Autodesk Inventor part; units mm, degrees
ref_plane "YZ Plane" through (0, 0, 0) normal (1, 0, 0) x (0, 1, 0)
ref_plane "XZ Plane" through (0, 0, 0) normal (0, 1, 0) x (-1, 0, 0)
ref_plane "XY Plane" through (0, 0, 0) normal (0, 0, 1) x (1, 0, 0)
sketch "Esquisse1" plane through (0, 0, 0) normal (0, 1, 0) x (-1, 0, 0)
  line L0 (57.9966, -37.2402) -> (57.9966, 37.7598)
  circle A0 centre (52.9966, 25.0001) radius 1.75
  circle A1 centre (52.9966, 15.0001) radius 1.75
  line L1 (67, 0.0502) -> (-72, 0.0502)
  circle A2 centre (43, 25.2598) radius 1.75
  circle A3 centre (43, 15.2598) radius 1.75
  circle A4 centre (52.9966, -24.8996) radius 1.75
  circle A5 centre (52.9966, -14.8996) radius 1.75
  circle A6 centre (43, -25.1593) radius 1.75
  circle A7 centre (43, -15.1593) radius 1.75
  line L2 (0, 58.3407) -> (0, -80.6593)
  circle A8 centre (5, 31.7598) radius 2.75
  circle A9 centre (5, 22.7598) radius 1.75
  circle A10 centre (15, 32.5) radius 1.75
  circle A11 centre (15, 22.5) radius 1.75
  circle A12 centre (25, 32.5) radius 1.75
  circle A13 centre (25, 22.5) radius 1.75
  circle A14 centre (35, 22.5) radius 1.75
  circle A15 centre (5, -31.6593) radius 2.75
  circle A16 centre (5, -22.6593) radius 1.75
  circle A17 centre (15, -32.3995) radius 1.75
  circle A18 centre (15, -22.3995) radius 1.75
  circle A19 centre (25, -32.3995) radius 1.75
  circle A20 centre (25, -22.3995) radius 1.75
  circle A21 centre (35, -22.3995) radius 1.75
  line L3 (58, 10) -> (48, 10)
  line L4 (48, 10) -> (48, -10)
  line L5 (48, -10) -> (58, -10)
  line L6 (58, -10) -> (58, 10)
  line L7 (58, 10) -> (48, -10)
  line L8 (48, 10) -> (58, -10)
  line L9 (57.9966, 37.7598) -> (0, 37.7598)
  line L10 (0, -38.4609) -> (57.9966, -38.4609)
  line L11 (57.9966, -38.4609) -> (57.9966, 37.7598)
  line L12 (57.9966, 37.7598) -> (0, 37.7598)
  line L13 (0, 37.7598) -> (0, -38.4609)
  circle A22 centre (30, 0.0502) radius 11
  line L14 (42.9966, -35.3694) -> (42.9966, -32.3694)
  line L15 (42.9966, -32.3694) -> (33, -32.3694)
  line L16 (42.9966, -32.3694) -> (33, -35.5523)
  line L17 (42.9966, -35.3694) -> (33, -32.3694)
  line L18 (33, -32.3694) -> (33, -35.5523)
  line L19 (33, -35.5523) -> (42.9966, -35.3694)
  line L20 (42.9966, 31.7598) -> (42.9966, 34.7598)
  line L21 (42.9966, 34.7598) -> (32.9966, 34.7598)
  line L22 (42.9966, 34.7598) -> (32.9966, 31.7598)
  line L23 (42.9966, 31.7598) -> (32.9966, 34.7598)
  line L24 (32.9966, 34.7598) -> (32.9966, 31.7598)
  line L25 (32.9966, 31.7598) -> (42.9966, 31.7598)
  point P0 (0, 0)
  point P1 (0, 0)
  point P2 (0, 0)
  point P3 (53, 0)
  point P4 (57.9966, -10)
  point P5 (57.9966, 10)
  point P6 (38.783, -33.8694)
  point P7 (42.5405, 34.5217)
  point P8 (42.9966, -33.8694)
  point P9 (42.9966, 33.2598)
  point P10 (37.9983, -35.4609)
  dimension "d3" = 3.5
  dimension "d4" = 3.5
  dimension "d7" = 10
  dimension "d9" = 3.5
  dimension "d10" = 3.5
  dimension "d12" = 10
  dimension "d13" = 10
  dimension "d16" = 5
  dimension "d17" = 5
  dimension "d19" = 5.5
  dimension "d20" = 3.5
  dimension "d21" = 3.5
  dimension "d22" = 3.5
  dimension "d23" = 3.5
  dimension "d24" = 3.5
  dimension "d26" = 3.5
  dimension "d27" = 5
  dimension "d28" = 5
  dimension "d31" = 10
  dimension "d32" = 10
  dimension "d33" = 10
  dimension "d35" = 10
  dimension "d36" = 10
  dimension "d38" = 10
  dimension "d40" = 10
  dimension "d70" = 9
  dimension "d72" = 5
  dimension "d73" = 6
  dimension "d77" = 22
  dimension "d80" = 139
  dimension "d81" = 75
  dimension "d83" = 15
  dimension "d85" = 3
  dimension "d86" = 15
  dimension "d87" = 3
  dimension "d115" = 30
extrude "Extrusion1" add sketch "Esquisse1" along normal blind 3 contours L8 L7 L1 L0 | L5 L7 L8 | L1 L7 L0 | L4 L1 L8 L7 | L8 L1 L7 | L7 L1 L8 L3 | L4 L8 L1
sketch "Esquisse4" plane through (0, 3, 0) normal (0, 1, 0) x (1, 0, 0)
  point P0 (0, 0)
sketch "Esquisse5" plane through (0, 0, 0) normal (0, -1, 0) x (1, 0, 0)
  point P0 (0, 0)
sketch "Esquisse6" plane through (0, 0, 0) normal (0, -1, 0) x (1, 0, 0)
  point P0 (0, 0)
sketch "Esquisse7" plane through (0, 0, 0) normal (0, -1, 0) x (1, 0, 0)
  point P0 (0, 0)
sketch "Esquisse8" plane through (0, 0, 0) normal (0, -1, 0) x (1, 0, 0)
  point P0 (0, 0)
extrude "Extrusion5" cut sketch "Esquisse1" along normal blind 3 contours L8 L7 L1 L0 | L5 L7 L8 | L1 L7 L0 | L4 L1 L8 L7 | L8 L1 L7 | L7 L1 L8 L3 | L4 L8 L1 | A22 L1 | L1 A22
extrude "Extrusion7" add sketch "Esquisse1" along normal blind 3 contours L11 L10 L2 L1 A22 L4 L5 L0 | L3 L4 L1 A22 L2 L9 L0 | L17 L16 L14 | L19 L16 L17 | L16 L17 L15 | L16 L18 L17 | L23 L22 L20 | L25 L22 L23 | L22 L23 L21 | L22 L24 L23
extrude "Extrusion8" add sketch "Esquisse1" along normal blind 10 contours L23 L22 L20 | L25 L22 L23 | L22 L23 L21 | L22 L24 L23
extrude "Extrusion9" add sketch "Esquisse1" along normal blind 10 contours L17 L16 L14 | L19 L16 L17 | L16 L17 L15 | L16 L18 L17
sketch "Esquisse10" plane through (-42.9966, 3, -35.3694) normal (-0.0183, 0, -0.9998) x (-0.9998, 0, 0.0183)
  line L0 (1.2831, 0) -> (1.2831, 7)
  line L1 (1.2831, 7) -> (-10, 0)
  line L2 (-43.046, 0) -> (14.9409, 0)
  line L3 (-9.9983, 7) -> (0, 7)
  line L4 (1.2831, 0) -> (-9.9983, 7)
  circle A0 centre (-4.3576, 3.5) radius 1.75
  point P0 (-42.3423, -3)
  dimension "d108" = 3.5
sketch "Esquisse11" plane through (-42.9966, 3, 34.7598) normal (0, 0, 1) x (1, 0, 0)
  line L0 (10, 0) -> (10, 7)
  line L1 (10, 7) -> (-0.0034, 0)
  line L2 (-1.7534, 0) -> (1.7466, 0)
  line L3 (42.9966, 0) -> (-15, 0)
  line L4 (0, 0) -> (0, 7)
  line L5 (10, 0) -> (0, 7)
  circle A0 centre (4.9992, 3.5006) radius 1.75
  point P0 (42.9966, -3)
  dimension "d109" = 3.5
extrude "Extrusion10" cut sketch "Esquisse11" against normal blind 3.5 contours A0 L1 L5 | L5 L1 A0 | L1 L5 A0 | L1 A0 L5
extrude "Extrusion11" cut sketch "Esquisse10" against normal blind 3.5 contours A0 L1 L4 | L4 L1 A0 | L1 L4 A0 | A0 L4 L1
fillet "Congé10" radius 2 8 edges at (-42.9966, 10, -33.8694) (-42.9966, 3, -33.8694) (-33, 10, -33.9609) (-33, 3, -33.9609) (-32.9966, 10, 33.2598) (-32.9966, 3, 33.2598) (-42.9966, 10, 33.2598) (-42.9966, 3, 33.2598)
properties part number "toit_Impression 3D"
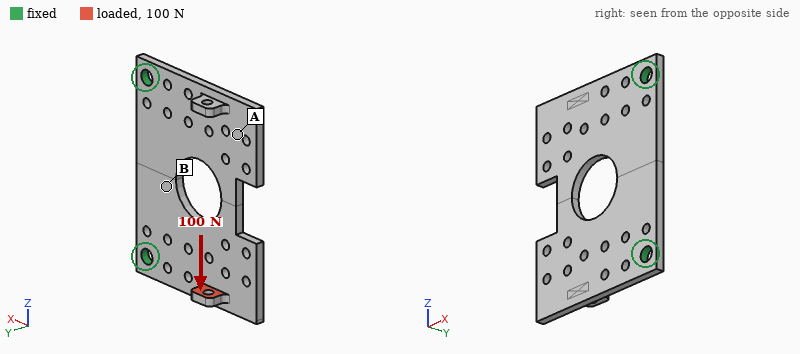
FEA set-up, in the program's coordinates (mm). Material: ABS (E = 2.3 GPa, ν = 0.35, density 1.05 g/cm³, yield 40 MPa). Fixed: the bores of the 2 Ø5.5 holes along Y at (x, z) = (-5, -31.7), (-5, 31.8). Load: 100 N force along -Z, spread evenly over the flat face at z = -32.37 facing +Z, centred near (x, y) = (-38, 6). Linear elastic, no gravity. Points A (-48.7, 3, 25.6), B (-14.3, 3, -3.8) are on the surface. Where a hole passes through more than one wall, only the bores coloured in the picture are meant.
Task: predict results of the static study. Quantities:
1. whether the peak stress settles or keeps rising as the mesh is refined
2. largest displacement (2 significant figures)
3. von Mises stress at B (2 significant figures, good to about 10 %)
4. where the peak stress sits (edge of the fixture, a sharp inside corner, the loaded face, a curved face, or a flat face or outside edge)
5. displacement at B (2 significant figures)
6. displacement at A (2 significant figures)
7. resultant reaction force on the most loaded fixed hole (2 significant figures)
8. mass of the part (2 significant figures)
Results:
keeps rising
0.97 mm
3.3 MPa
a sharp inside corner
0.20 mm
0.54 mm
69 N
12 g
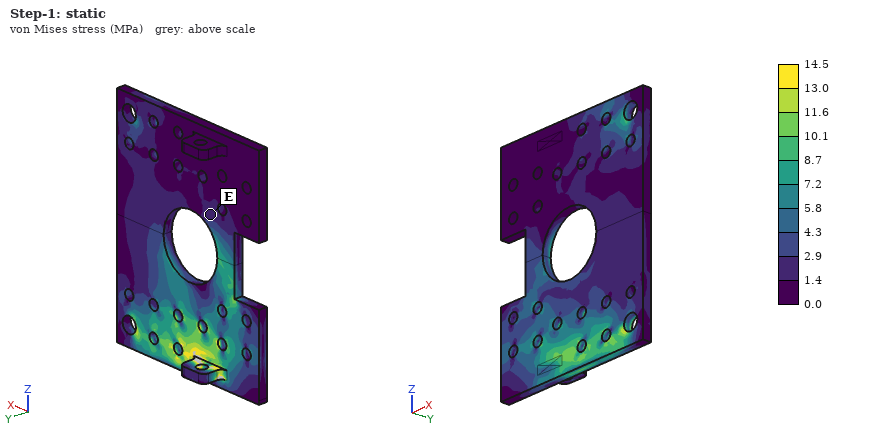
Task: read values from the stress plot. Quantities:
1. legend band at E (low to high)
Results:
1.4 to 2.9 MPa
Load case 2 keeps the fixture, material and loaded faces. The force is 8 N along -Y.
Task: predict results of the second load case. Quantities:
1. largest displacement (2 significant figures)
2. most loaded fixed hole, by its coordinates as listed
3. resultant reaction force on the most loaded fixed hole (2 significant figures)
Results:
1.1 mm
(-5, -31.7)
8.0 N
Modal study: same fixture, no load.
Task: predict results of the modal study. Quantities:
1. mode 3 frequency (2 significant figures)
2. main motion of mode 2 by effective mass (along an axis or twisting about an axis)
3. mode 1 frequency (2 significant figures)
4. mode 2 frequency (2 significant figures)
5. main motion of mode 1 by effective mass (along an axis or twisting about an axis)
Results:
850 Hz
twisting about X
220 Hz
400 Hz
along Y
